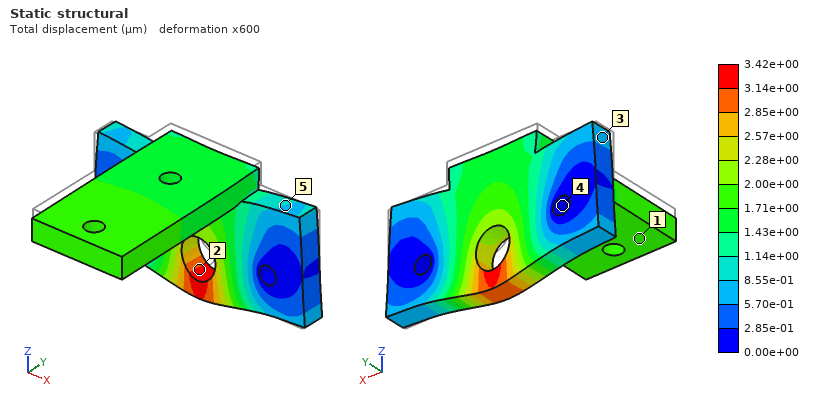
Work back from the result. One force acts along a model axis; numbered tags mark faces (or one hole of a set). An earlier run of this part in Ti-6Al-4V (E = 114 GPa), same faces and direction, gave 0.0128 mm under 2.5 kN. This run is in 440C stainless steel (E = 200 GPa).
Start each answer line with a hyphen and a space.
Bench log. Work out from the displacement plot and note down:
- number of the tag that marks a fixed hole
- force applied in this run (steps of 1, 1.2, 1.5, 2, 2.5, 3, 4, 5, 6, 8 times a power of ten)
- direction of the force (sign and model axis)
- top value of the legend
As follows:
- 4
- 1.2 kN
- -Z
- 3.42e+00 µm
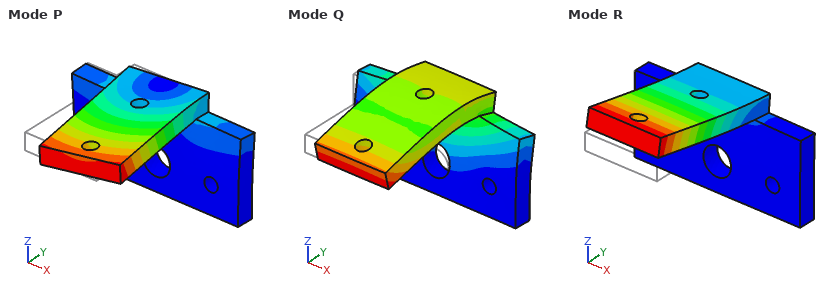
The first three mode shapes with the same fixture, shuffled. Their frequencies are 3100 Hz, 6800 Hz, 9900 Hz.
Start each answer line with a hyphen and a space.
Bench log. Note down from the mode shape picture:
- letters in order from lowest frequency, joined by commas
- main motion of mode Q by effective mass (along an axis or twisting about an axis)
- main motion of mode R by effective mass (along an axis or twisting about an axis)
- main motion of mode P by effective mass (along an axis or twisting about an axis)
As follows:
- R, P, Q
- along Y
- along Z
- along X
